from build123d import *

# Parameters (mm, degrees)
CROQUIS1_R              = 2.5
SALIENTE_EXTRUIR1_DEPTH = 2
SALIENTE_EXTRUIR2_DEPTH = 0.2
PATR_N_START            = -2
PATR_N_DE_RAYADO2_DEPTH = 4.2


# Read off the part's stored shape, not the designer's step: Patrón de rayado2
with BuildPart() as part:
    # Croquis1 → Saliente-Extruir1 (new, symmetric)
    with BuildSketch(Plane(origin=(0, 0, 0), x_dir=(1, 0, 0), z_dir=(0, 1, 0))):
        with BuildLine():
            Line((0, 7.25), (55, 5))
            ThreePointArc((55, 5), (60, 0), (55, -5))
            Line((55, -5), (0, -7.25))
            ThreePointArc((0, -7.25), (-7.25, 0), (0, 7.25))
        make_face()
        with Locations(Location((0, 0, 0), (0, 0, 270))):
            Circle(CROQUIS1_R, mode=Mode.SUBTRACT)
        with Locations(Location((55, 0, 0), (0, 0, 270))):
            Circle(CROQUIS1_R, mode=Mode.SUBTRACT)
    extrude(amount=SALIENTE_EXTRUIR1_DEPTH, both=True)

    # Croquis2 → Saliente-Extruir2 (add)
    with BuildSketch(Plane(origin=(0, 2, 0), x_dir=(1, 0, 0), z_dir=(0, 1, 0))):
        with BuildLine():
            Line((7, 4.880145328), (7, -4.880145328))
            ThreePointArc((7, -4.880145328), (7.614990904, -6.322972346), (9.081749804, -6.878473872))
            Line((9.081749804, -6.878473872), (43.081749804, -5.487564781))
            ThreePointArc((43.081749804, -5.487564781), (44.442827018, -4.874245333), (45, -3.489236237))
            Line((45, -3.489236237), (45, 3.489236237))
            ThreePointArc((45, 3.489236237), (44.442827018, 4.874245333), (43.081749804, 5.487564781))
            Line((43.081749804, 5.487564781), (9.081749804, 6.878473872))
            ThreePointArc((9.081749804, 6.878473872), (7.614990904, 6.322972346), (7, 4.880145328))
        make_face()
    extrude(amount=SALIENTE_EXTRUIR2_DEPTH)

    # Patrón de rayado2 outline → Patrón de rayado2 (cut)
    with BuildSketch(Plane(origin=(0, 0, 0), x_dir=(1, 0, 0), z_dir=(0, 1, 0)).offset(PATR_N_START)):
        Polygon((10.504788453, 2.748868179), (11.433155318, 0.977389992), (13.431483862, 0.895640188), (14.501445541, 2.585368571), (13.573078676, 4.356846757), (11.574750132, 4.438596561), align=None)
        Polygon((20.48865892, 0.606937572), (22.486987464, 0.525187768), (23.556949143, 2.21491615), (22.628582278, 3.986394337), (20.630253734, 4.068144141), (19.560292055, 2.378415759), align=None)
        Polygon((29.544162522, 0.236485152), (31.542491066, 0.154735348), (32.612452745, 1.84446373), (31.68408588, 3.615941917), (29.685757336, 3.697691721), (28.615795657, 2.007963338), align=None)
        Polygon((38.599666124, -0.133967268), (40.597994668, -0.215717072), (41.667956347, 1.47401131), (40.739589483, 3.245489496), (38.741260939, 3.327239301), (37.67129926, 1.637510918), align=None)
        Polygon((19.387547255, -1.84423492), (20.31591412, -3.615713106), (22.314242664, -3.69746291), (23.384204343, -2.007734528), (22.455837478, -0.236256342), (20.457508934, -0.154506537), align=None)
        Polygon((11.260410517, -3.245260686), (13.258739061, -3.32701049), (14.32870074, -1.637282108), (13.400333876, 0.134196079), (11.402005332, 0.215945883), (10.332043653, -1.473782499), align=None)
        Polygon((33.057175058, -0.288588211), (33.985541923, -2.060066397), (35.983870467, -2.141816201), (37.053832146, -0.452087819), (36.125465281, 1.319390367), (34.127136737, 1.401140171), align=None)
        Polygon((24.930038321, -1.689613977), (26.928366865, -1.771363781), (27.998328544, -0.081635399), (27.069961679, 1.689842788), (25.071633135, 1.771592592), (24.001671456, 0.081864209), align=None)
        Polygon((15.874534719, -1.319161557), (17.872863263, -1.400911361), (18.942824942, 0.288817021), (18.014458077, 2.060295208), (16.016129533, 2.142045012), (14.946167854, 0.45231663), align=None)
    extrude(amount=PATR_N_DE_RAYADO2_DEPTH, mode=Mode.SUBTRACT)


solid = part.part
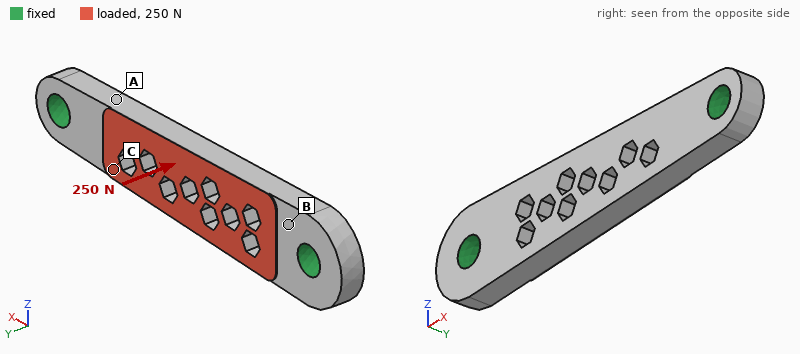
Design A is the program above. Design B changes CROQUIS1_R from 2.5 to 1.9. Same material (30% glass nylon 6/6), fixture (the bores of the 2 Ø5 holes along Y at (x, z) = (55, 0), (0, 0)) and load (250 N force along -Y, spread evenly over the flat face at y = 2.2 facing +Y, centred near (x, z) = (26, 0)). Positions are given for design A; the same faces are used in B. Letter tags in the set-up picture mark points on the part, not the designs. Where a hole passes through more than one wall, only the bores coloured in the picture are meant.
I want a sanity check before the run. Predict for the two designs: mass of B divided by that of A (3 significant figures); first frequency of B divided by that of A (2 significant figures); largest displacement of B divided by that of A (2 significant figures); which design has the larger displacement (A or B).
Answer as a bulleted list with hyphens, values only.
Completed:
- 1.02
- 0.94
- 1.1
- B
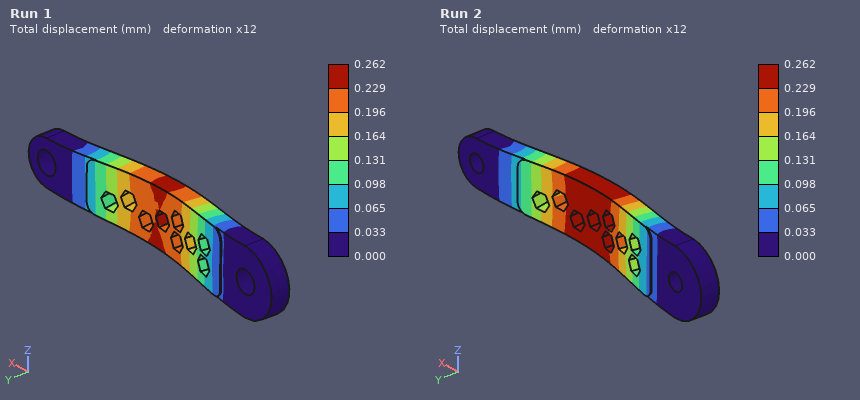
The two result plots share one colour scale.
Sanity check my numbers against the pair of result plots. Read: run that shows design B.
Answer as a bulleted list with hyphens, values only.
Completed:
- Run 2
